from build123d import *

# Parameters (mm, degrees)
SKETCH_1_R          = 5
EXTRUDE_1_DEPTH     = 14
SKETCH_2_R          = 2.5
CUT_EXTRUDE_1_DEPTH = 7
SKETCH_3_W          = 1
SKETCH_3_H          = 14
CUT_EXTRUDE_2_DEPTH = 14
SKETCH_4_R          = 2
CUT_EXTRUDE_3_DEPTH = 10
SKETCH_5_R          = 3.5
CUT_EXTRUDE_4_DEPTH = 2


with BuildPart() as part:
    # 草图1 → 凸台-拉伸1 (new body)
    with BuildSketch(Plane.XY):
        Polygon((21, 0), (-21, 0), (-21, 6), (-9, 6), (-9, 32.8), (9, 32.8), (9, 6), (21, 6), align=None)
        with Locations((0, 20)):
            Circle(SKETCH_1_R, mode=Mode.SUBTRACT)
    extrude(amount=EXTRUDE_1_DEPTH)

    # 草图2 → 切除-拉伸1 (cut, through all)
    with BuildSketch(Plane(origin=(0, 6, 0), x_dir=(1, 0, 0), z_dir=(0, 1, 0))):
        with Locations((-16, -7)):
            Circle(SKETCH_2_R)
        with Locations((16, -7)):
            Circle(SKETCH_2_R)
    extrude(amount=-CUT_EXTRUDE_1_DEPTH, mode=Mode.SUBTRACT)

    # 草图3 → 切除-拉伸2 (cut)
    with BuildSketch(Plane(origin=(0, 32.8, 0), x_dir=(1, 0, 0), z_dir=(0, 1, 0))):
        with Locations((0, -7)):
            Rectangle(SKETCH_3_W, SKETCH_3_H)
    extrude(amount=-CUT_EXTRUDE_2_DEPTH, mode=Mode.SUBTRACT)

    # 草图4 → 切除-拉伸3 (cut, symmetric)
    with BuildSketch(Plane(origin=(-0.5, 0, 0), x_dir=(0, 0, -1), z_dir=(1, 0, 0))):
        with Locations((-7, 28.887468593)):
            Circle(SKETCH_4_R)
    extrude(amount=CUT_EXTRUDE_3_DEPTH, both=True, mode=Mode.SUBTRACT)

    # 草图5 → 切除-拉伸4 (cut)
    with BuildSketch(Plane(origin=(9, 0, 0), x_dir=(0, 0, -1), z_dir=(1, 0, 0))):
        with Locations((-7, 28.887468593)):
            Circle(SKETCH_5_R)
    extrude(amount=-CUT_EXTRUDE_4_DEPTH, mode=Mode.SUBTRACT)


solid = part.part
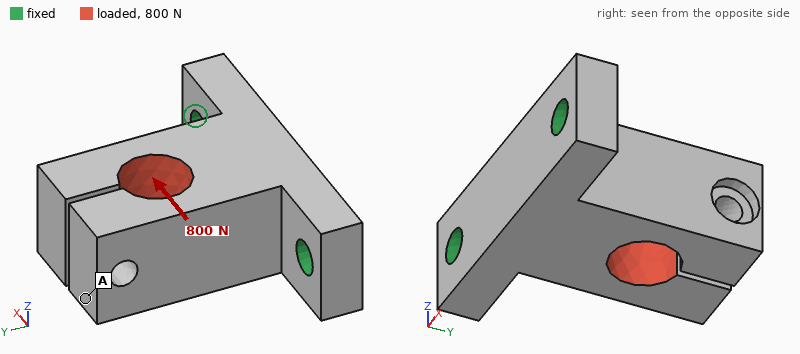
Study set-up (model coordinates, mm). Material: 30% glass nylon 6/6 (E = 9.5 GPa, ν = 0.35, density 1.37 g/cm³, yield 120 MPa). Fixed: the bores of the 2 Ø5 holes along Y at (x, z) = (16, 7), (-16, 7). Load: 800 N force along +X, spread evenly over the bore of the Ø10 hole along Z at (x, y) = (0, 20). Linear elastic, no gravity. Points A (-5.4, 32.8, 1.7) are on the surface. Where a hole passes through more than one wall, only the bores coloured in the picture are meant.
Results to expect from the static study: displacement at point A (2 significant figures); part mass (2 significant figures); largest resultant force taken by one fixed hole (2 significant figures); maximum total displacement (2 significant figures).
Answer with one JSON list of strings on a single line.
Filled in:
["0.24 mm", "12 g", "680 N", "0.25 mm"]
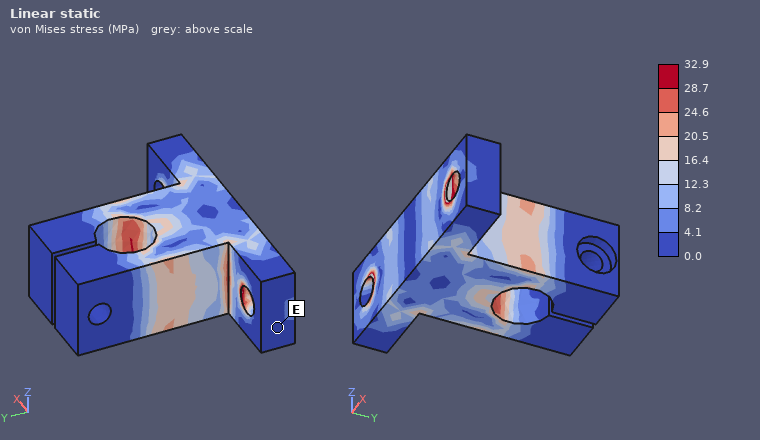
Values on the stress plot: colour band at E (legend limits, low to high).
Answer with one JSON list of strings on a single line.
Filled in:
["0.0 to 4.1 MPa"]
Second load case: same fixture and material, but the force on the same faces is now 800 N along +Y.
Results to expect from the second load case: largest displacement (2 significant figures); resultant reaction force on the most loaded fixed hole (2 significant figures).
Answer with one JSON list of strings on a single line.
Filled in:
["0.12 mm", "430 N"]
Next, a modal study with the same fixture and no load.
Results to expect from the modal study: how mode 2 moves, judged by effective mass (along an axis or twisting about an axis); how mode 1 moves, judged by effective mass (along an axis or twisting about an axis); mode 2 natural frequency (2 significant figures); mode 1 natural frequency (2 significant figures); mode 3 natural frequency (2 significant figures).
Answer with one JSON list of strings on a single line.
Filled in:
["along X", "along Z", "3600 Hz", "2700 Hz", "4000 Hz"]
